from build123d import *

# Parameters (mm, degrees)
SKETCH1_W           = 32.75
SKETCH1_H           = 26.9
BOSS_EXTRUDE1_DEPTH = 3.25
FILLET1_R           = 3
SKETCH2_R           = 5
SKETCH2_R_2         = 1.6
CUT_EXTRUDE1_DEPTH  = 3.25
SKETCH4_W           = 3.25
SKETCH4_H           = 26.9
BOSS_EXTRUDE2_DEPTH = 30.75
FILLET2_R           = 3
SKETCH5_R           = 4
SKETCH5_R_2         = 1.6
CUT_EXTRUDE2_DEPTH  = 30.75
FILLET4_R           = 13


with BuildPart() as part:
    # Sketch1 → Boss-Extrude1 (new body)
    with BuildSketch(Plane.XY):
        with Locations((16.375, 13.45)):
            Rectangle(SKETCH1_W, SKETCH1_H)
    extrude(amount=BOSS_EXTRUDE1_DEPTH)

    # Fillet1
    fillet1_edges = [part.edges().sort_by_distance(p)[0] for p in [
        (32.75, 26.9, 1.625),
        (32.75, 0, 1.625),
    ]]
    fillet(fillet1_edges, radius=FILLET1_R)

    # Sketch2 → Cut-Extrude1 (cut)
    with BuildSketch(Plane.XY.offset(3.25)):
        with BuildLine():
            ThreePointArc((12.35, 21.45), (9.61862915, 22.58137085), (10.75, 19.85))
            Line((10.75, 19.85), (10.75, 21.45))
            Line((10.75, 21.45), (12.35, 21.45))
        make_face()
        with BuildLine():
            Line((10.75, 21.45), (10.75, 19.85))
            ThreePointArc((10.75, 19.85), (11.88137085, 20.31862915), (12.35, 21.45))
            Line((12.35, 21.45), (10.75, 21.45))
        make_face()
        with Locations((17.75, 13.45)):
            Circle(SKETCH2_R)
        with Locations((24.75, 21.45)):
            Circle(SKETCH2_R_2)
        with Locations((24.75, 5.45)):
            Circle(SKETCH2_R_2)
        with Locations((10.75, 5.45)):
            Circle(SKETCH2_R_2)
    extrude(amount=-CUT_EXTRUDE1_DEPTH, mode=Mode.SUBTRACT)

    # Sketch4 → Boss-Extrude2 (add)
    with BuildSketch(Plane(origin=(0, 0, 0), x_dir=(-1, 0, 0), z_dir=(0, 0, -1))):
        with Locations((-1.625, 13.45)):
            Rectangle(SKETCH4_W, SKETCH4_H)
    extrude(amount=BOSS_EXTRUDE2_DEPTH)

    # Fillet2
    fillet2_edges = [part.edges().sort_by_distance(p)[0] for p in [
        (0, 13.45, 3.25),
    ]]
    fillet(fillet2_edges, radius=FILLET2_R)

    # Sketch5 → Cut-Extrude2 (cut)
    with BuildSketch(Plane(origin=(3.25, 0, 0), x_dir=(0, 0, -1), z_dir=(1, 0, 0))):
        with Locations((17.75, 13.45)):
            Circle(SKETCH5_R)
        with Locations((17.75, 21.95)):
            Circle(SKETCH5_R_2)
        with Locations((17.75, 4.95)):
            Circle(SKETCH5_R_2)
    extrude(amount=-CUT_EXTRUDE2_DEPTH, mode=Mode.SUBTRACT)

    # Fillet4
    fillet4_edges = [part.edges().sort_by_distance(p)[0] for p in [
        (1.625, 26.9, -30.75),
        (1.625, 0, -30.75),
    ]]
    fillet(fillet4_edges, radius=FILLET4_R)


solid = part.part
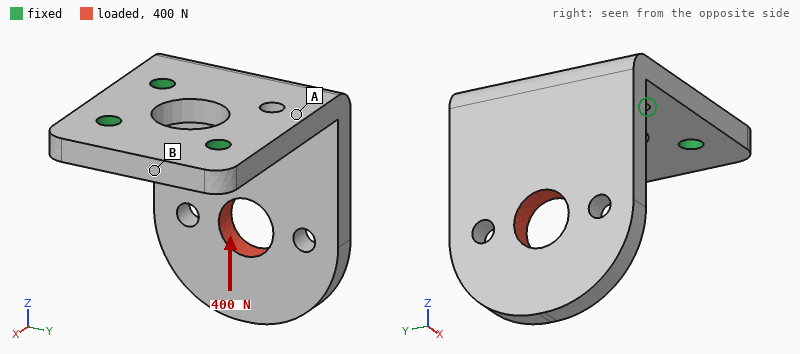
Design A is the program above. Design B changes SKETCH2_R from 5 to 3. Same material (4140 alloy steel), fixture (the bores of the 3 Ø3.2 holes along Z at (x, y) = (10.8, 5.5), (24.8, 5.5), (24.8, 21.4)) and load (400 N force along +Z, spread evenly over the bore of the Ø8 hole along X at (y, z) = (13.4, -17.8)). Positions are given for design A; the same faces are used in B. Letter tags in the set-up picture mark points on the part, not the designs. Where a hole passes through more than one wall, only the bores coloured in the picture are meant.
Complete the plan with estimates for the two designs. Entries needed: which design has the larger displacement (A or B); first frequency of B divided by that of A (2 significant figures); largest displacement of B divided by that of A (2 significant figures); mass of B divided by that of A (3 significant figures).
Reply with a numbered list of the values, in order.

1. A
2. 1.0
3. 0.92
4. 1.03
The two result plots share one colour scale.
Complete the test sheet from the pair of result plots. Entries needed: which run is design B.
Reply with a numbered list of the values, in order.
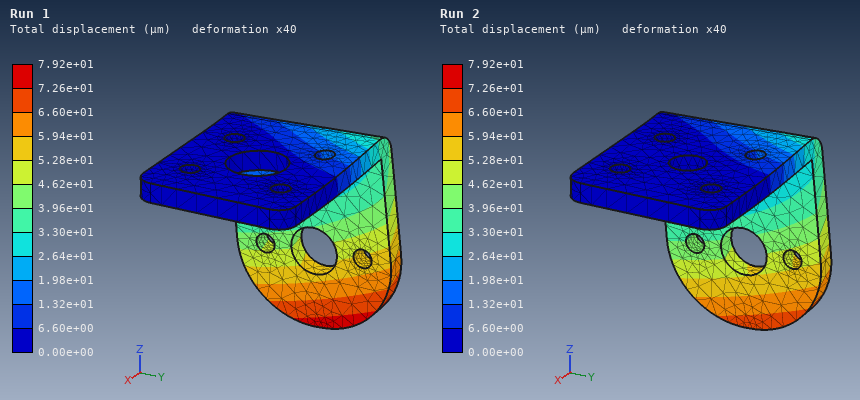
1. Run 2
